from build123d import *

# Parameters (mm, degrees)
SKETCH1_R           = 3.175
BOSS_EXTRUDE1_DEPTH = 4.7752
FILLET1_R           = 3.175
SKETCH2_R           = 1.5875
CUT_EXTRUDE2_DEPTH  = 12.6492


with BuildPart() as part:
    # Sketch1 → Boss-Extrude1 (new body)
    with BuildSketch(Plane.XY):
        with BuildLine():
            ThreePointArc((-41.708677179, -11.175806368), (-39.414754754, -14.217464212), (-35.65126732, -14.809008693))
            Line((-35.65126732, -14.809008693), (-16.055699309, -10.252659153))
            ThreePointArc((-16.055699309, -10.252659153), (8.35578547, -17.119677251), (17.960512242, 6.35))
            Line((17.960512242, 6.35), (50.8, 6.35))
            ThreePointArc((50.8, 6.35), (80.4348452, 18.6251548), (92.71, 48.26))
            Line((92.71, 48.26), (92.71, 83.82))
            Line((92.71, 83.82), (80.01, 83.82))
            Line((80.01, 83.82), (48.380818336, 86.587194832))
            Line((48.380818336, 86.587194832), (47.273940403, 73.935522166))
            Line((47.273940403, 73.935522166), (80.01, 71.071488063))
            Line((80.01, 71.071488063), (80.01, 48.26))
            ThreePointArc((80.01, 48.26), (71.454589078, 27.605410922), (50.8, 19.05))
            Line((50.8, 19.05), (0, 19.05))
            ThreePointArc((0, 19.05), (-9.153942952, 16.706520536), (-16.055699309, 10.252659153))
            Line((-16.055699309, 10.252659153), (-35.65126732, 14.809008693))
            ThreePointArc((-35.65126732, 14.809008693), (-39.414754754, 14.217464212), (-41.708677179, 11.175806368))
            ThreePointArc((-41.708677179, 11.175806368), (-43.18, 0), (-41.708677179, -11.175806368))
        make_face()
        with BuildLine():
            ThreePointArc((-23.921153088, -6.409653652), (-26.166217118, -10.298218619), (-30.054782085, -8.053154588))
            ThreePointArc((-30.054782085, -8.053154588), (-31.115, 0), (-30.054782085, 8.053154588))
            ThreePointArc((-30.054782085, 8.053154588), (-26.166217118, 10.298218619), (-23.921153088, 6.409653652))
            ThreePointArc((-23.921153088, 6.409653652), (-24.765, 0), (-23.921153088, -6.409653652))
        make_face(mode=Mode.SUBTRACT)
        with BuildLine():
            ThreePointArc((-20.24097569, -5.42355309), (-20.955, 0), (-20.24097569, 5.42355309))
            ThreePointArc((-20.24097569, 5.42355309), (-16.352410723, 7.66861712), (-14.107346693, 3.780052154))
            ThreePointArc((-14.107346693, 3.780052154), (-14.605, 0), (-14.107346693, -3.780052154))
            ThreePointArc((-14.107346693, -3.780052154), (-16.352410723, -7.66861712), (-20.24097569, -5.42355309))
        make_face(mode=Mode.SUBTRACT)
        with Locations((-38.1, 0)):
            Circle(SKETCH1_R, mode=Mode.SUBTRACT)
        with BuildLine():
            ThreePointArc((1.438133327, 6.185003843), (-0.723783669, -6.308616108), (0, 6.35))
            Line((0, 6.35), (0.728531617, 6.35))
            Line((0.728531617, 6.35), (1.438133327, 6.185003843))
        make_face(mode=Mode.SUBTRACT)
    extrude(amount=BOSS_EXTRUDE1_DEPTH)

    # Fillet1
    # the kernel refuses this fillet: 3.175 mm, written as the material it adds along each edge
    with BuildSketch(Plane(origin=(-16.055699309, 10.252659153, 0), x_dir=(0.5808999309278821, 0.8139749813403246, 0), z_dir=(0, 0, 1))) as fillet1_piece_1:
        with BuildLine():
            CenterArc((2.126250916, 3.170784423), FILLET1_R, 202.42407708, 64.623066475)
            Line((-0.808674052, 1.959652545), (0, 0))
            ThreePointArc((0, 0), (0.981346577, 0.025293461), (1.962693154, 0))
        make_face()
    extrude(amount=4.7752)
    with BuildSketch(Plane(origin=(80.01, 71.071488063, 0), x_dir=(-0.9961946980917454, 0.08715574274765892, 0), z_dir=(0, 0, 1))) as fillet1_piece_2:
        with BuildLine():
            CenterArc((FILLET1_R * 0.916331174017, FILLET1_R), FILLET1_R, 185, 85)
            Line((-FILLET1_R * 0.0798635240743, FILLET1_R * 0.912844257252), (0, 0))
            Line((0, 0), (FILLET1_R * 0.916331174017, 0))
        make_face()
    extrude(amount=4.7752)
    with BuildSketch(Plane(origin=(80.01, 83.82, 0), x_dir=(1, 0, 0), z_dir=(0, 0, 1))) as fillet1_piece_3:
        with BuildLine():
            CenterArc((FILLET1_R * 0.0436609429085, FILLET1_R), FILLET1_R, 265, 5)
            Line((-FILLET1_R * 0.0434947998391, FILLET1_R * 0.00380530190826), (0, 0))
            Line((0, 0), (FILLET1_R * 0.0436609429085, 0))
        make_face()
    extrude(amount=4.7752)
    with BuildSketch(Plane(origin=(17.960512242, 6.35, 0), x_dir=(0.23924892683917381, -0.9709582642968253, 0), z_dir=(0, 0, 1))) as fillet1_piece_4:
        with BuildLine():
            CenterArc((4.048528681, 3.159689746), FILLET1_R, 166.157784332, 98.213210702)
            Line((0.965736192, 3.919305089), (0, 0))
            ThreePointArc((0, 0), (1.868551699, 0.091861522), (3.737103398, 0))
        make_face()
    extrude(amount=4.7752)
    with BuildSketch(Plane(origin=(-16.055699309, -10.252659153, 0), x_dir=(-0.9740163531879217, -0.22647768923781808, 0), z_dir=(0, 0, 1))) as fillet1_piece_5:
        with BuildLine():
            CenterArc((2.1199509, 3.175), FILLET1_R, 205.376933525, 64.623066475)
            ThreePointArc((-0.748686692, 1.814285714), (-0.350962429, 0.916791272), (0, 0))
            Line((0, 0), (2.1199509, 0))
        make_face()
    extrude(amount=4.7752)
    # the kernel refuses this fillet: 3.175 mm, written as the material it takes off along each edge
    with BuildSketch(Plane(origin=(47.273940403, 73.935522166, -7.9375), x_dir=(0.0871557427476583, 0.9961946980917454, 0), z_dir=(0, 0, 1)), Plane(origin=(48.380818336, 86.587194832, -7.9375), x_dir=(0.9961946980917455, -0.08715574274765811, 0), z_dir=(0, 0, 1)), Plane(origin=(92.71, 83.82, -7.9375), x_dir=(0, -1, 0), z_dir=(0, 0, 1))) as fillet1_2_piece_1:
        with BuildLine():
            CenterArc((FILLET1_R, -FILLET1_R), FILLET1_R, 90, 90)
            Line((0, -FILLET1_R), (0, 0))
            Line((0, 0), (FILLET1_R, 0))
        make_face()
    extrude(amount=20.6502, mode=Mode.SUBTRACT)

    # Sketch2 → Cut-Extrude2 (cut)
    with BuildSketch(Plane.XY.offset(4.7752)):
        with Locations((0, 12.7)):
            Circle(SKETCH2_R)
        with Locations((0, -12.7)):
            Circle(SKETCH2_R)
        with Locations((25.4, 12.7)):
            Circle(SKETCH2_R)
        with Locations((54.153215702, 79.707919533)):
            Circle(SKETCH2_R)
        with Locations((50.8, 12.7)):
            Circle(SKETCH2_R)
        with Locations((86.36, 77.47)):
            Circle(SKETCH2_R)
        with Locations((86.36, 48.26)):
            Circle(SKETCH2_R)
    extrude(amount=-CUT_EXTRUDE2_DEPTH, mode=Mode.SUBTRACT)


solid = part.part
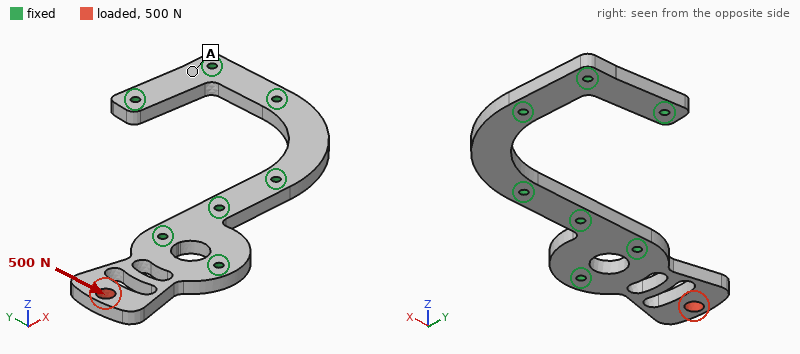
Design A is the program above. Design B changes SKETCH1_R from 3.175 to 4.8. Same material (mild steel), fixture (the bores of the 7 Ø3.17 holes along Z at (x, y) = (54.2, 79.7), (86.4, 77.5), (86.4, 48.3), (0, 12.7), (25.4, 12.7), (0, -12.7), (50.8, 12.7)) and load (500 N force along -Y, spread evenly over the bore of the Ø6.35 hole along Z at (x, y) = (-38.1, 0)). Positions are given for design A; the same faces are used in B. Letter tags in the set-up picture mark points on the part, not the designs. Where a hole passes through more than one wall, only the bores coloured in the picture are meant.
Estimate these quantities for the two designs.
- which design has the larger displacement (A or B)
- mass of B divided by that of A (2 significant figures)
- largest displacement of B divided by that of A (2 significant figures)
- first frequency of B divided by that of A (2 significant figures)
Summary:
B
0.99
1.2
1.1
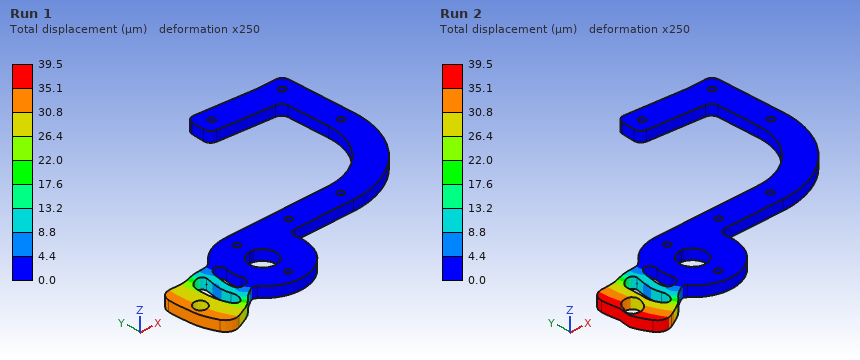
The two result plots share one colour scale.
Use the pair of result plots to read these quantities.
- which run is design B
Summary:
Run 2
